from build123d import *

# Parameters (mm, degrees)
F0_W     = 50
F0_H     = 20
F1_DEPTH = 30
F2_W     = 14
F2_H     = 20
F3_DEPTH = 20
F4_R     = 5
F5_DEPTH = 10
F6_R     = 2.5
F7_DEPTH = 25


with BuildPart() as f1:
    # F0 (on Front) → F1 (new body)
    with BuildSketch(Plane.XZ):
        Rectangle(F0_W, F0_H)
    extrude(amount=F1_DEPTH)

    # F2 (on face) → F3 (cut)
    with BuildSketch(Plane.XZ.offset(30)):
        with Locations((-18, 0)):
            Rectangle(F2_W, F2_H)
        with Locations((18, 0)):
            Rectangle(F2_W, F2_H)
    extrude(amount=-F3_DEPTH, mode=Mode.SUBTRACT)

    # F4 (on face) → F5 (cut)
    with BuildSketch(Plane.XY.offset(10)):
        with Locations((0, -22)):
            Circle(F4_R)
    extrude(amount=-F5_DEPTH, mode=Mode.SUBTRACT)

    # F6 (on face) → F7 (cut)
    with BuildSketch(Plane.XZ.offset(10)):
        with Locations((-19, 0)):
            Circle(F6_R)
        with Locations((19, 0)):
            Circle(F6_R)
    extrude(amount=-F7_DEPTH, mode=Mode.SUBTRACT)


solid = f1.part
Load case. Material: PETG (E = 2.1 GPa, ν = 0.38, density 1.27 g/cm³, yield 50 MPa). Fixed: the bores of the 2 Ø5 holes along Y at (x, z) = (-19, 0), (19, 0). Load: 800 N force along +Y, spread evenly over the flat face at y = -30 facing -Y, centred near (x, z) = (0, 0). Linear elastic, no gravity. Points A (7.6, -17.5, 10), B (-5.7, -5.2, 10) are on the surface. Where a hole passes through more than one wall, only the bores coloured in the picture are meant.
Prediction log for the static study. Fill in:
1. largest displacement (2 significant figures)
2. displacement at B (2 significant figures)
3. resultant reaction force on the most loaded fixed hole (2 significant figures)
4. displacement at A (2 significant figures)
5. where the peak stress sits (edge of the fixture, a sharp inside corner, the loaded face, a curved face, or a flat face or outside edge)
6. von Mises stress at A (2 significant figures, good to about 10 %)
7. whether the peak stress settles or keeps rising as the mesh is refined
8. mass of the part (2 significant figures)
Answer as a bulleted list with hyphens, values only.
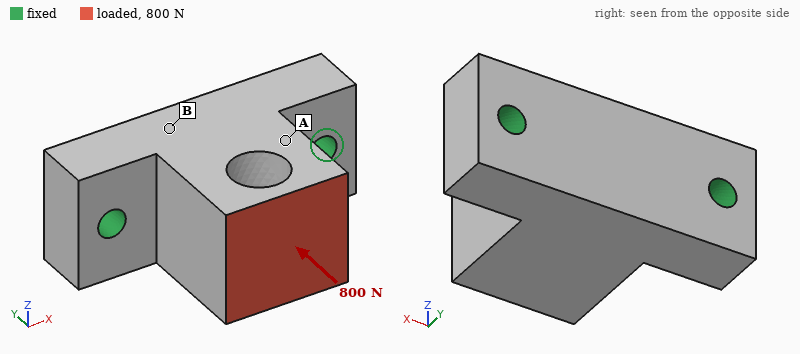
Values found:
- 0.10 mm
- 0.056 mm
- 420 N
- 0.061 mm
- edge of the fixture
- 3.7 MPa
- keeps rising
- 22 g
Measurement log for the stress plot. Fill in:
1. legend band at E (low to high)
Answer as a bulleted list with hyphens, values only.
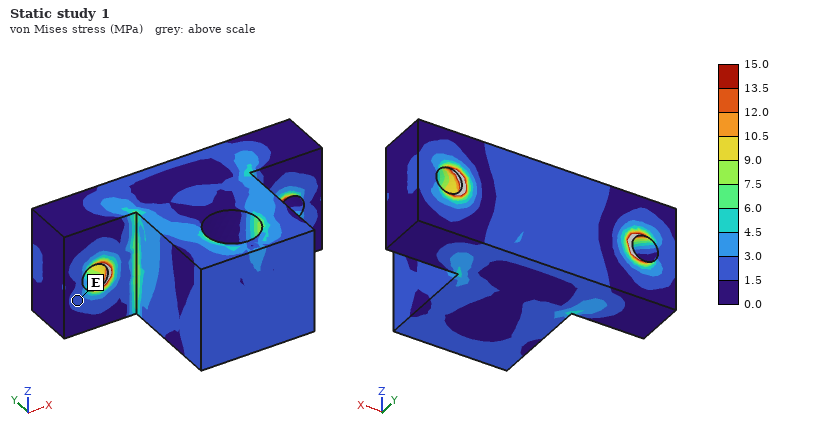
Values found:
- 1.5 to 3.0 MPa
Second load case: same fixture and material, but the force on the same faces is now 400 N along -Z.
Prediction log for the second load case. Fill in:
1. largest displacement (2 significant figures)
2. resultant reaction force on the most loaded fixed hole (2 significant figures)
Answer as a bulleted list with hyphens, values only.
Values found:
- 0.51 mm
- 200 N
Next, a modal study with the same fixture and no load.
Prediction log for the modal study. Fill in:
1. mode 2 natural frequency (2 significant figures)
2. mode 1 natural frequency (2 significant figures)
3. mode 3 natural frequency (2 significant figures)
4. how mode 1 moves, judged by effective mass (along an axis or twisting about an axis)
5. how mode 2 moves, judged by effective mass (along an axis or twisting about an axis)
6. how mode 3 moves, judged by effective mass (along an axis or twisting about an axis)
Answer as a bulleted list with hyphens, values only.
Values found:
- 4100 Hz
- 2100 Hz
- 4700 Hz
- along Z
- along X
- along Y
